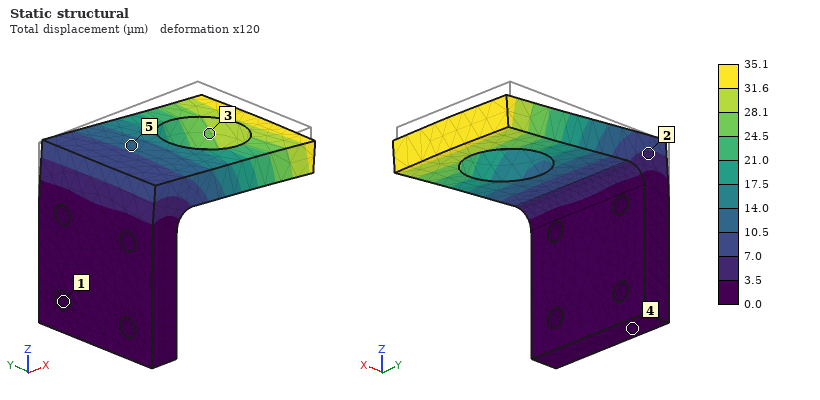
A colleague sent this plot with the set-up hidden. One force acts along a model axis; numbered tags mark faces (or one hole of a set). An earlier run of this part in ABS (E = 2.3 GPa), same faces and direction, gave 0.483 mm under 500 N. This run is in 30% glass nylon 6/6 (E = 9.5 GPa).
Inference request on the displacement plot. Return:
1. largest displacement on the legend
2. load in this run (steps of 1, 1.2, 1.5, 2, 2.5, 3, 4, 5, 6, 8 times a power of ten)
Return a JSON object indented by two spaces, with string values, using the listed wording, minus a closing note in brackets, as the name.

{
  "largest displacement on the legend": "35.1 µm",
  "load in this run": "150 N"
}
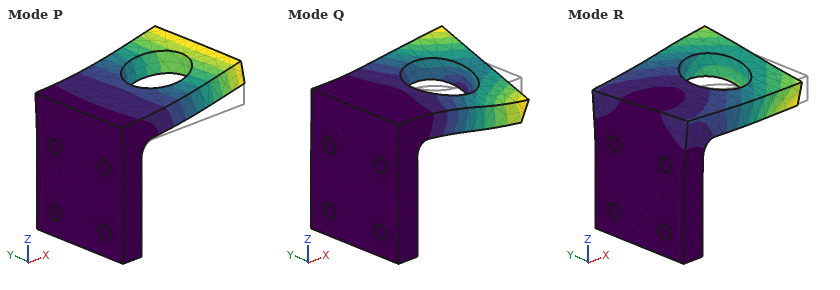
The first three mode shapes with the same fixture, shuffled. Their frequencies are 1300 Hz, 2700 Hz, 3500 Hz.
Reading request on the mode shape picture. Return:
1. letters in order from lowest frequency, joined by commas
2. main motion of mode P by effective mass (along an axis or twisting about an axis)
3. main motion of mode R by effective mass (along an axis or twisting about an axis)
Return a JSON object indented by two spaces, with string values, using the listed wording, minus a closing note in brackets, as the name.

{
  "letters in order from lowest frequency, joined by commas": "P, R, Q",
  "main motion of mode P by effective mass": "along Z",
  "main motion of mode R by effective mass": "along Y"
}
